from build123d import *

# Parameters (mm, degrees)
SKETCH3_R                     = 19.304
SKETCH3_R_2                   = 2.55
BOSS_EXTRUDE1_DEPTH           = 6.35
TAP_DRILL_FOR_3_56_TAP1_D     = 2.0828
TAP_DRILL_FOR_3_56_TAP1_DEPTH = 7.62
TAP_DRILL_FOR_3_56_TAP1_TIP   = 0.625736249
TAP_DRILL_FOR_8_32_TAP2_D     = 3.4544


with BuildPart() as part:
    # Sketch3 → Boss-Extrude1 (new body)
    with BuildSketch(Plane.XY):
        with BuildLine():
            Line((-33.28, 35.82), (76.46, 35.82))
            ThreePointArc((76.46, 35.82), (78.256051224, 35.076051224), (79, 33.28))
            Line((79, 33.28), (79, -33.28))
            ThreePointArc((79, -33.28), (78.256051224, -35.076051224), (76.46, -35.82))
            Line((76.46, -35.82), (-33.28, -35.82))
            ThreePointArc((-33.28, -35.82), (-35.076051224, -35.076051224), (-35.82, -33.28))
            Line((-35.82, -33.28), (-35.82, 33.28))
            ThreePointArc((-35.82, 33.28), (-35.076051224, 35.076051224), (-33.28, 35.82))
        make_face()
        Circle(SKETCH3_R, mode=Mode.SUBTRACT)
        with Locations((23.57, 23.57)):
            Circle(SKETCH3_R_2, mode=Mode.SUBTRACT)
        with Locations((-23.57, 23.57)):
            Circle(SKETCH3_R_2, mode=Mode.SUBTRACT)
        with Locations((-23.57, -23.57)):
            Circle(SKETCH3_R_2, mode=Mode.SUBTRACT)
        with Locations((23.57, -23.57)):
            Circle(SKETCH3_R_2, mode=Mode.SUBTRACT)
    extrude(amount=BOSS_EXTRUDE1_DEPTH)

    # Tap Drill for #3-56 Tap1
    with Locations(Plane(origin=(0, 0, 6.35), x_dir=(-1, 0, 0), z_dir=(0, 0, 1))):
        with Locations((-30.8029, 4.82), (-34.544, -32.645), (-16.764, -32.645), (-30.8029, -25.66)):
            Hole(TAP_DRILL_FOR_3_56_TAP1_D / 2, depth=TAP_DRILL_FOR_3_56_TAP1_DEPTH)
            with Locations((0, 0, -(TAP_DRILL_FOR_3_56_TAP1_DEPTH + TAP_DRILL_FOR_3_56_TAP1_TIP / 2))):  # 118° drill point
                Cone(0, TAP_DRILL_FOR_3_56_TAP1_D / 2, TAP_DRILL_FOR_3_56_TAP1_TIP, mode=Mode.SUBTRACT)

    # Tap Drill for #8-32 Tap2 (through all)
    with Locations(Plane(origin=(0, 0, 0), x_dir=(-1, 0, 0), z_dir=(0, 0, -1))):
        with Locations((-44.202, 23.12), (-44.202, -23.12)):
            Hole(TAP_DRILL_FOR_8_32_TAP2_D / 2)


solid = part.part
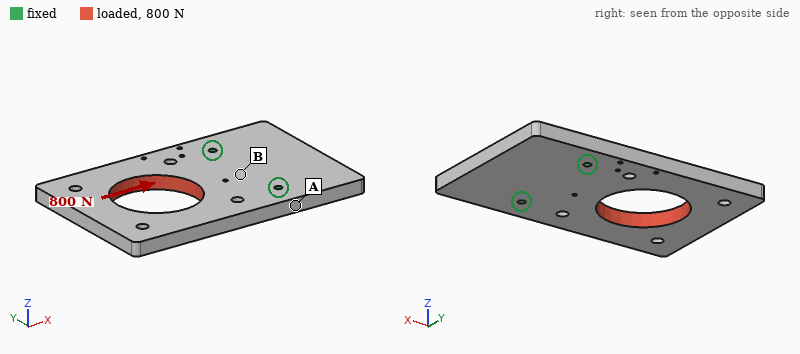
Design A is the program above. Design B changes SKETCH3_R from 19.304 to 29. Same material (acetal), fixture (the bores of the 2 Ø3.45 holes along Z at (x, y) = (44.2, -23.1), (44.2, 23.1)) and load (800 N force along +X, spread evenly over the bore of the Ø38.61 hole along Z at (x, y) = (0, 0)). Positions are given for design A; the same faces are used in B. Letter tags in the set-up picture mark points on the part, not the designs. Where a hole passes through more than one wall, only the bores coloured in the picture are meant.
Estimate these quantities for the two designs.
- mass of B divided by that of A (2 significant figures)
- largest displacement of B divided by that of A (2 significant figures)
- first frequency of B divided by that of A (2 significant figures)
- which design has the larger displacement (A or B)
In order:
0.79
4.5
0.91
B
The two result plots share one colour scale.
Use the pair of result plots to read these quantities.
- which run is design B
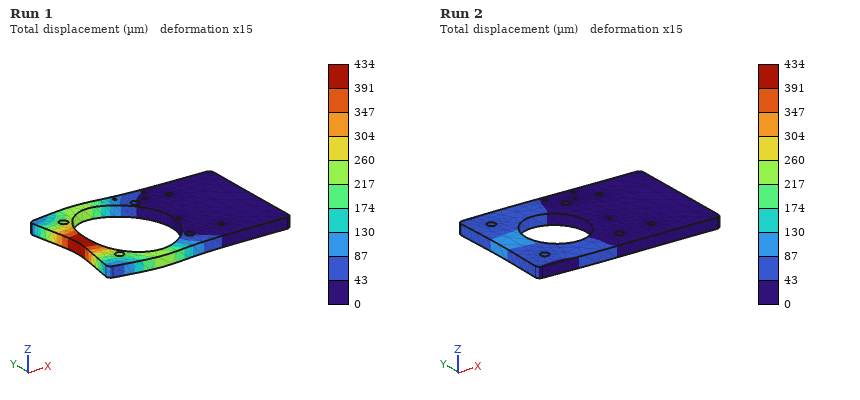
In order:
Run 1
